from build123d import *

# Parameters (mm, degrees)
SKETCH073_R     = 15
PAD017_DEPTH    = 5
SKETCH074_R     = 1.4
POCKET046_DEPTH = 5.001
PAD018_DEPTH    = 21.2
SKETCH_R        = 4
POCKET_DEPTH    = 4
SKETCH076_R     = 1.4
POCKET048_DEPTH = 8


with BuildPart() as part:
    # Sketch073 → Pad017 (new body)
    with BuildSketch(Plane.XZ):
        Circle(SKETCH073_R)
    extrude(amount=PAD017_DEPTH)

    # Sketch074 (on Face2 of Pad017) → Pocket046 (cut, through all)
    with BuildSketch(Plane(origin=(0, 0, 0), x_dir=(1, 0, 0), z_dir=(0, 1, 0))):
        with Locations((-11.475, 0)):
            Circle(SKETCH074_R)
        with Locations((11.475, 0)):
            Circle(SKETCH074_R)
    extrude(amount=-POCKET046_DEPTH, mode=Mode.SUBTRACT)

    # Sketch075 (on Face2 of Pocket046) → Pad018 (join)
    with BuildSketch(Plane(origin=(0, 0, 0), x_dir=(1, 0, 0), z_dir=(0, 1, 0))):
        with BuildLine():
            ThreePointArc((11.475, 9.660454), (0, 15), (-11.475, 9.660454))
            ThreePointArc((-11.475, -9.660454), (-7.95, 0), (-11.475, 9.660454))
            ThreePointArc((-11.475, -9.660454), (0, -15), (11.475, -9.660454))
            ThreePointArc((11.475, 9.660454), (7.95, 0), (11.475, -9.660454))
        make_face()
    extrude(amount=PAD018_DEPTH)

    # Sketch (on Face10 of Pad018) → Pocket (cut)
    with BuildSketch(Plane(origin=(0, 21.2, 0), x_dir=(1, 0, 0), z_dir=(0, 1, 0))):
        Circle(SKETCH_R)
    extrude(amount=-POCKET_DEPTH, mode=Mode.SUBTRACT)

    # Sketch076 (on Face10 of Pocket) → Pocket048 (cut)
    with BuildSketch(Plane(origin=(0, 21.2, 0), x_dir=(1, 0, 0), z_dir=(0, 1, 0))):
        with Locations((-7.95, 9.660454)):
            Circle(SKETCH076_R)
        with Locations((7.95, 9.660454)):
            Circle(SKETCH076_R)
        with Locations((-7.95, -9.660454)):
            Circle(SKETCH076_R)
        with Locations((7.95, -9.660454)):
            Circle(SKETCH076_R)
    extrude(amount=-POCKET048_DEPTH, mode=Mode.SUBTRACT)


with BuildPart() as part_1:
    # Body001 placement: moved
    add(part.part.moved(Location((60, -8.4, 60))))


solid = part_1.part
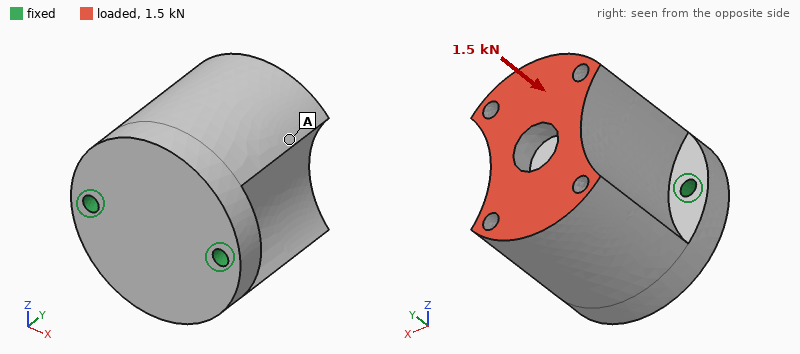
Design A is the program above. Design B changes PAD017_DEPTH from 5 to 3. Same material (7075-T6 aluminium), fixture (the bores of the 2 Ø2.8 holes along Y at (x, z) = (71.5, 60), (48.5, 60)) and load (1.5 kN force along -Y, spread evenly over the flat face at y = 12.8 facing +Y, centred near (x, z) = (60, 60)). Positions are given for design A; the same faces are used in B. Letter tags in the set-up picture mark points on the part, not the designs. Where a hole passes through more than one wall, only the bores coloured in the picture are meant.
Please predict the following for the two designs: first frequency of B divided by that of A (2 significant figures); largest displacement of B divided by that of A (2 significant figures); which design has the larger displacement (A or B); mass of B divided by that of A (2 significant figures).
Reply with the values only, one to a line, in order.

0.63
1.8
B
0.90
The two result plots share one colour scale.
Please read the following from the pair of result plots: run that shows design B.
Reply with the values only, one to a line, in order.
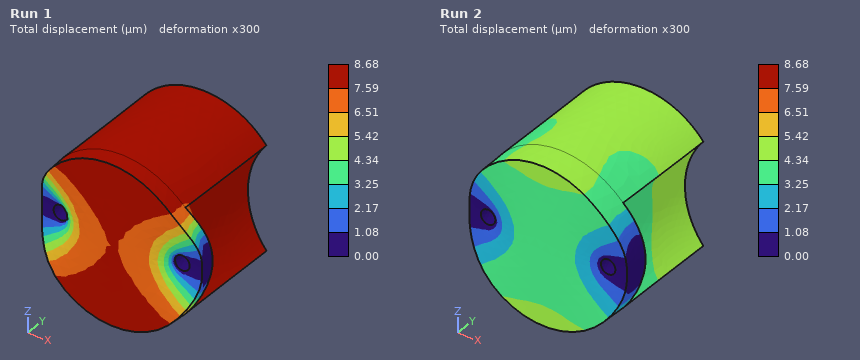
Run 1
